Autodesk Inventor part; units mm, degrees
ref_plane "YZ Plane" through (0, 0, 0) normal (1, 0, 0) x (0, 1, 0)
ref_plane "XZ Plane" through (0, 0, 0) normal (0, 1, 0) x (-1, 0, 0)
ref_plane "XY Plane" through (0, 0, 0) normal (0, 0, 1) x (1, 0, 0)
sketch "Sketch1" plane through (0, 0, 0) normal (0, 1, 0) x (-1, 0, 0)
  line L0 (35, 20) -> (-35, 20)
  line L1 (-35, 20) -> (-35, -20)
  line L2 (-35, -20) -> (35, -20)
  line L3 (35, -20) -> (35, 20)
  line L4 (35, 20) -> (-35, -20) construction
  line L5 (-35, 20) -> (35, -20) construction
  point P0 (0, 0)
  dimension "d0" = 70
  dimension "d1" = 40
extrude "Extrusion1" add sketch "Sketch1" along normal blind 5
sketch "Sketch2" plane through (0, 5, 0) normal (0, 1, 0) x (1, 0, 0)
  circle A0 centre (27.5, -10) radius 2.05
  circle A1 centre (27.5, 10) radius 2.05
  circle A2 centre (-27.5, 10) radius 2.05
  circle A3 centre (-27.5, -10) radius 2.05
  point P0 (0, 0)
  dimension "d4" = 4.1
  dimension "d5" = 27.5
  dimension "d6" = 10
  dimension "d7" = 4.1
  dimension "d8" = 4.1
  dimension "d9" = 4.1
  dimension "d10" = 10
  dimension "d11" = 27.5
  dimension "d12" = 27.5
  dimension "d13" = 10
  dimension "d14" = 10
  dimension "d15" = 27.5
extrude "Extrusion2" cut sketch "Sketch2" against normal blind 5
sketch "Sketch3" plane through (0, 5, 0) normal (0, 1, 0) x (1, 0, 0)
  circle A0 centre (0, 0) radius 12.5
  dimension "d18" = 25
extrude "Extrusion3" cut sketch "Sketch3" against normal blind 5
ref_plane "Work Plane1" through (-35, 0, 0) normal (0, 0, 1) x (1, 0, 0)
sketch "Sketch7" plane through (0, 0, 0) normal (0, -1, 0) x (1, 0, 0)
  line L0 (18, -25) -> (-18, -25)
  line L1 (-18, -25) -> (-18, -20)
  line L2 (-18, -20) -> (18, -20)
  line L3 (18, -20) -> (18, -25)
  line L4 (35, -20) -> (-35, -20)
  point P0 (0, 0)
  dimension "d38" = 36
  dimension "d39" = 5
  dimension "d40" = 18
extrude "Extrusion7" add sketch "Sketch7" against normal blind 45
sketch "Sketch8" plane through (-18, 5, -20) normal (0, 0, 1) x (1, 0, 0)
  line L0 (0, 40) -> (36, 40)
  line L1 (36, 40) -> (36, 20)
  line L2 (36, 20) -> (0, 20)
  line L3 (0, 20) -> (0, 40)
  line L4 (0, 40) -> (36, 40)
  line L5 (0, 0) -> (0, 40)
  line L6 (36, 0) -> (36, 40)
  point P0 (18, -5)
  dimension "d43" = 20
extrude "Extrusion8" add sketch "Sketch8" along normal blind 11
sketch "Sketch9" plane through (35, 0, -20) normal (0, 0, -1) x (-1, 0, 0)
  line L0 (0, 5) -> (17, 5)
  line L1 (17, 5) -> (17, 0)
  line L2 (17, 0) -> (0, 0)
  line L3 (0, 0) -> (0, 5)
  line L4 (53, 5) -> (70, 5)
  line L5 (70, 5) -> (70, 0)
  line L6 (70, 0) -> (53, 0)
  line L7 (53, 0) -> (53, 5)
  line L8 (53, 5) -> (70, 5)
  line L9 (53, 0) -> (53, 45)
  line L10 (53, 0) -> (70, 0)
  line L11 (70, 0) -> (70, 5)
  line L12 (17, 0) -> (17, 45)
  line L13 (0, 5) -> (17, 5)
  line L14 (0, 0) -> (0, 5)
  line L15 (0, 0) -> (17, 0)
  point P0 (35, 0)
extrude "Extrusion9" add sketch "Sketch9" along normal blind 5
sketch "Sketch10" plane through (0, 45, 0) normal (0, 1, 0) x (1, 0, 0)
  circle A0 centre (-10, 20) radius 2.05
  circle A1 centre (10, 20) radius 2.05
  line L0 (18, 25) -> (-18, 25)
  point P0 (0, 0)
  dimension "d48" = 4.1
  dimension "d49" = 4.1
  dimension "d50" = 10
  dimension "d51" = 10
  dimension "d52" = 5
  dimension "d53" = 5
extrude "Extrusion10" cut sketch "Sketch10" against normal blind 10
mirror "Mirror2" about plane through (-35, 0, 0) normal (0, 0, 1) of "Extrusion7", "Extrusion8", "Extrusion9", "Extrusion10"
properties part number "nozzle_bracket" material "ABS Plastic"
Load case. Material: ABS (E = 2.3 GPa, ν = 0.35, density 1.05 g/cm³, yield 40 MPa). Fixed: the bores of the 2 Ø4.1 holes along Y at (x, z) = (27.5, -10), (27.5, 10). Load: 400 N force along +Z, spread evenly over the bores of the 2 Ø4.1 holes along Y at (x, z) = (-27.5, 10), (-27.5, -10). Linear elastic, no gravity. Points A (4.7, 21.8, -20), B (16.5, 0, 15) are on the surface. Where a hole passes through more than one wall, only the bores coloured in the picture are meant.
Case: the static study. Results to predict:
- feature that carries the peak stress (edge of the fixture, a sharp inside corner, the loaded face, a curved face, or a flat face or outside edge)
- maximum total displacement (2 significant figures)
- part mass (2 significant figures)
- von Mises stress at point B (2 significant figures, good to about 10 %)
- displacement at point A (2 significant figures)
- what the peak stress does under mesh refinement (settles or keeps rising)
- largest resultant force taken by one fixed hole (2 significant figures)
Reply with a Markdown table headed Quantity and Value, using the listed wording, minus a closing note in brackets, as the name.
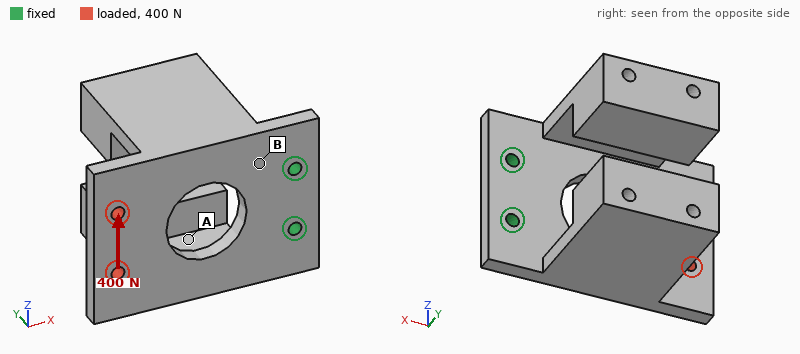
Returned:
| Quantity | Value |
|---|---|
| feature that carries the peak stress | edge of the fixture |
| maximum total displacement | 1.0 mm |
| part mass | 47 g |
| von Mises stress at point B | 6.5 MPa |
| displacement at point A | 0.38 mm |
| what the peak stress does under mesh refinement | keeps rising |
| largest resultant force taken by one fixed hole | 940 N |
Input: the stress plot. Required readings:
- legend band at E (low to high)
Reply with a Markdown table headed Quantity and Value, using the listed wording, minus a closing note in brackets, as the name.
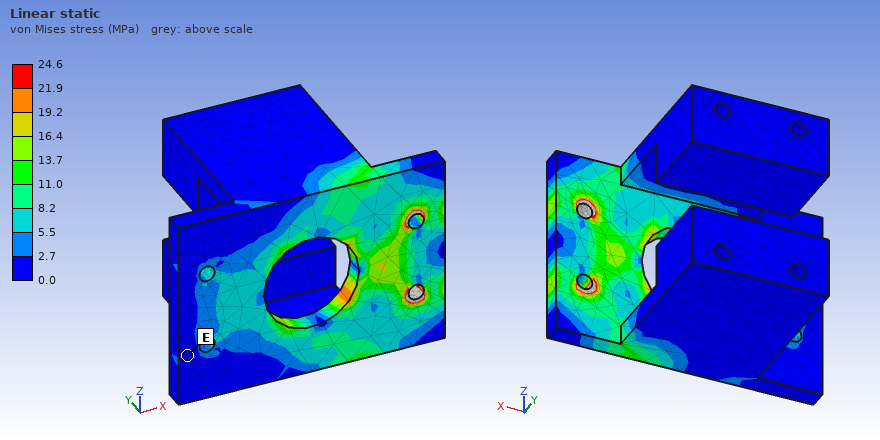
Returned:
| Quantity | Value |
|---|---|
| legend band at E | 0.0 to 2.7 MPa |
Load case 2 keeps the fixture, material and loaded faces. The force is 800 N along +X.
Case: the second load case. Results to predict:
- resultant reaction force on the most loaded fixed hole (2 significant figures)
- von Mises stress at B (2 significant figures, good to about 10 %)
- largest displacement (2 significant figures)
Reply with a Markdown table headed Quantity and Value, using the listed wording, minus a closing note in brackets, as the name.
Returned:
| Quantity | Value |
|---|---|
| resultant reaction force on the most loaded fixed hole | 410 N |
| von Mises stress at B | 7.3 MPa |
| largest displacement | 0.23 mm |
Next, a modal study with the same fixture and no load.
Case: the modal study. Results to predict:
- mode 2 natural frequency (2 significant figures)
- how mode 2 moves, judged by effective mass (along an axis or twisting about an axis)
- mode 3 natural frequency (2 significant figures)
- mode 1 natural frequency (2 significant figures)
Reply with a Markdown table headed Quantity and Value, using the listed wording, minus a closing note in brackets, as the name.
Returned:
| Quantity | Value |
|---|---|
| mode 2 natural frequency | 200 Hz |
| how mode 2 moves, judged by effective mass | along Z |
| mode 3 natural frequency | 250 Hz |
| mode 1 natural frequency | 170 Hz |
